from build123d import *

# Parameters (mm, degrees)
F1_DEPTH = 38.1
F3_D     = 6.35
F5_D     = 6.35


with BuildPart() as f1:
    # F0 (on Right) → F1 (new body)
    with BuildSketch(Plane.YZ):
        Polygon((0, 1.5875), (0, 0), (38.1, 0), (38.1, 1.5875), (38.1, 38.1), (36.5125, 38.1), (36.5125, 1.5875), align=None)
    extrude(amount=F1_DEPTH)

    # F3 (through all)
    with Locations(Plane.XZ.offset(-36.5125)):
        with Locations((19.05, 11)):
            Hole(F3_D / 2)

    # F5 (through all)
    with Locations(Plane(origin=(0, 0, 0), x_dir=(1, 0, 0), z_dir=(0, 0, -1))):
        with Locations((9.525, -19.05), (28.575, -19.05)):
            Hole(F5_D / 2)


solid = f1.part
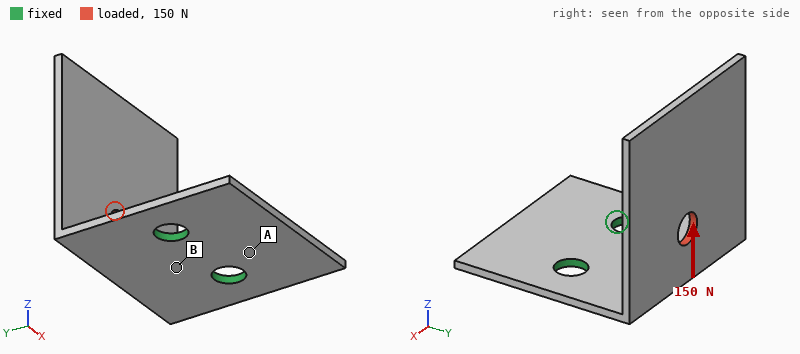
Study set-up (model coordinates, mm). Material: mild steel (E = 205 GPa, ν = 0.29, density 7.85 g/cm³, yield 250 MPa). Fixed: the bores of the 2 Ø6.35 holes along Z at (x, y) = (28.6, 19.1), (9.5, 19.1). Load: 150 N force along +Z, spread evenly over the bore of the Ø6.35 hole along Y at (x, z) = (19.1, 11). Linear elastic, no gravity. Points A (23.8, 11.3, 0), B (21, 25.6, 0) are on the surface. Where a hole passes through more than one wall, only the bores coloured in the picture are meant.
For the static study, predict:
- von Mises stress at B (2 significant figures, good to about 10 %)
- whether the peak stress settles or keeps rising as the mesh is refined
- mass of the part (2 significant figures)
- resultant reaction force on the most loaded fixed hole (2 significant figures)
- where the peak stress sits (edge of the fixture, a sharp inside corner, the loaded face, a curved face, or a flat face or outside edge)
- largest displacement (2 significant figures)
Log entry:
92 MPa
keeps rising
34 g
75 N
edge of the fixture
0.28 mm
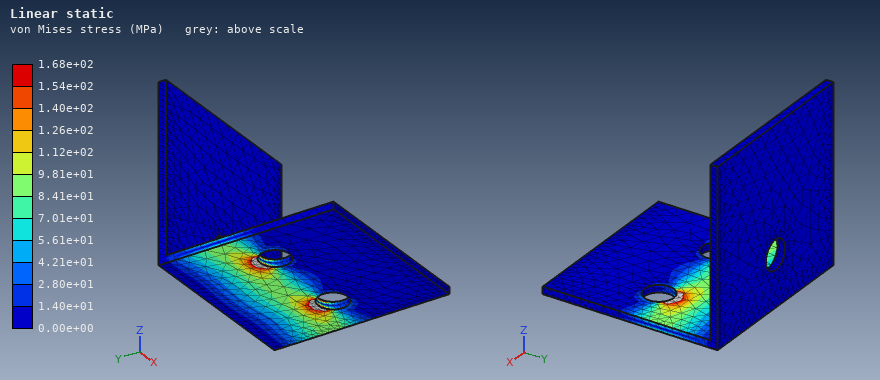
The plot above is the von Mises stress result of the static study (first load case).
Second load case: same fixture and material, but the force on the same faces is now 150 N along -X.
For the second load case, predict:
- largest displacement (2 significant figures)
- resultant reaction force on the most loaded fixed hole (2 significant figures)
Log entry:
0.10 mm
140 N
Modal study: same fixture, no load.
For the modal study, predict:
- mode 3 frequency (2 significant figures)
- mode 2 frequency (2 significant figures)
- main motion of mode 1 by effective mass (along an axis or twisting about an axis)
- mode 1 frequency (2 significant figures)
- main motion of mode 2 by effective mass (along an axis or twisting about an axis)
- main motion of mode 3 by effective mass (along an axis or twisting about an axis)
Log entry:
2200 Hz
1200 Hz
along Y
560 Hz
along X
along Z
